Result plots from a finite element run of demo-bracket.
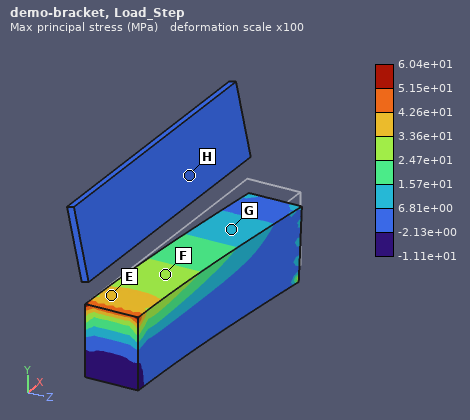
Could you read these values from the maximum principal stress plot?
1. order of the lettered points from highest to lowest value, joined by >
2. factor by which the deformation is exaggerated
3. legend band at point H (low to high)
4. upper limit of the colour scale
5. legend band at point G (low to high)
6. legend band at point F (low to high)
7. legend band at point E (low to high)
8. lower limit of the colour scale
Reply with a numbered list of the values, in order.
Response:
1. E > F > G > H
2. 100
3. -2.13e+00 to 6.81e+00 MPa
4. 6.04e+01 MPa
5. 6.81e+00 to 1.57e+01 MPa
6. 2.47e+01 to 3.36e+01 MPa
7. 3.36e+01 to 4.26e+01 MPa
8. -1.11e+01 MPa
